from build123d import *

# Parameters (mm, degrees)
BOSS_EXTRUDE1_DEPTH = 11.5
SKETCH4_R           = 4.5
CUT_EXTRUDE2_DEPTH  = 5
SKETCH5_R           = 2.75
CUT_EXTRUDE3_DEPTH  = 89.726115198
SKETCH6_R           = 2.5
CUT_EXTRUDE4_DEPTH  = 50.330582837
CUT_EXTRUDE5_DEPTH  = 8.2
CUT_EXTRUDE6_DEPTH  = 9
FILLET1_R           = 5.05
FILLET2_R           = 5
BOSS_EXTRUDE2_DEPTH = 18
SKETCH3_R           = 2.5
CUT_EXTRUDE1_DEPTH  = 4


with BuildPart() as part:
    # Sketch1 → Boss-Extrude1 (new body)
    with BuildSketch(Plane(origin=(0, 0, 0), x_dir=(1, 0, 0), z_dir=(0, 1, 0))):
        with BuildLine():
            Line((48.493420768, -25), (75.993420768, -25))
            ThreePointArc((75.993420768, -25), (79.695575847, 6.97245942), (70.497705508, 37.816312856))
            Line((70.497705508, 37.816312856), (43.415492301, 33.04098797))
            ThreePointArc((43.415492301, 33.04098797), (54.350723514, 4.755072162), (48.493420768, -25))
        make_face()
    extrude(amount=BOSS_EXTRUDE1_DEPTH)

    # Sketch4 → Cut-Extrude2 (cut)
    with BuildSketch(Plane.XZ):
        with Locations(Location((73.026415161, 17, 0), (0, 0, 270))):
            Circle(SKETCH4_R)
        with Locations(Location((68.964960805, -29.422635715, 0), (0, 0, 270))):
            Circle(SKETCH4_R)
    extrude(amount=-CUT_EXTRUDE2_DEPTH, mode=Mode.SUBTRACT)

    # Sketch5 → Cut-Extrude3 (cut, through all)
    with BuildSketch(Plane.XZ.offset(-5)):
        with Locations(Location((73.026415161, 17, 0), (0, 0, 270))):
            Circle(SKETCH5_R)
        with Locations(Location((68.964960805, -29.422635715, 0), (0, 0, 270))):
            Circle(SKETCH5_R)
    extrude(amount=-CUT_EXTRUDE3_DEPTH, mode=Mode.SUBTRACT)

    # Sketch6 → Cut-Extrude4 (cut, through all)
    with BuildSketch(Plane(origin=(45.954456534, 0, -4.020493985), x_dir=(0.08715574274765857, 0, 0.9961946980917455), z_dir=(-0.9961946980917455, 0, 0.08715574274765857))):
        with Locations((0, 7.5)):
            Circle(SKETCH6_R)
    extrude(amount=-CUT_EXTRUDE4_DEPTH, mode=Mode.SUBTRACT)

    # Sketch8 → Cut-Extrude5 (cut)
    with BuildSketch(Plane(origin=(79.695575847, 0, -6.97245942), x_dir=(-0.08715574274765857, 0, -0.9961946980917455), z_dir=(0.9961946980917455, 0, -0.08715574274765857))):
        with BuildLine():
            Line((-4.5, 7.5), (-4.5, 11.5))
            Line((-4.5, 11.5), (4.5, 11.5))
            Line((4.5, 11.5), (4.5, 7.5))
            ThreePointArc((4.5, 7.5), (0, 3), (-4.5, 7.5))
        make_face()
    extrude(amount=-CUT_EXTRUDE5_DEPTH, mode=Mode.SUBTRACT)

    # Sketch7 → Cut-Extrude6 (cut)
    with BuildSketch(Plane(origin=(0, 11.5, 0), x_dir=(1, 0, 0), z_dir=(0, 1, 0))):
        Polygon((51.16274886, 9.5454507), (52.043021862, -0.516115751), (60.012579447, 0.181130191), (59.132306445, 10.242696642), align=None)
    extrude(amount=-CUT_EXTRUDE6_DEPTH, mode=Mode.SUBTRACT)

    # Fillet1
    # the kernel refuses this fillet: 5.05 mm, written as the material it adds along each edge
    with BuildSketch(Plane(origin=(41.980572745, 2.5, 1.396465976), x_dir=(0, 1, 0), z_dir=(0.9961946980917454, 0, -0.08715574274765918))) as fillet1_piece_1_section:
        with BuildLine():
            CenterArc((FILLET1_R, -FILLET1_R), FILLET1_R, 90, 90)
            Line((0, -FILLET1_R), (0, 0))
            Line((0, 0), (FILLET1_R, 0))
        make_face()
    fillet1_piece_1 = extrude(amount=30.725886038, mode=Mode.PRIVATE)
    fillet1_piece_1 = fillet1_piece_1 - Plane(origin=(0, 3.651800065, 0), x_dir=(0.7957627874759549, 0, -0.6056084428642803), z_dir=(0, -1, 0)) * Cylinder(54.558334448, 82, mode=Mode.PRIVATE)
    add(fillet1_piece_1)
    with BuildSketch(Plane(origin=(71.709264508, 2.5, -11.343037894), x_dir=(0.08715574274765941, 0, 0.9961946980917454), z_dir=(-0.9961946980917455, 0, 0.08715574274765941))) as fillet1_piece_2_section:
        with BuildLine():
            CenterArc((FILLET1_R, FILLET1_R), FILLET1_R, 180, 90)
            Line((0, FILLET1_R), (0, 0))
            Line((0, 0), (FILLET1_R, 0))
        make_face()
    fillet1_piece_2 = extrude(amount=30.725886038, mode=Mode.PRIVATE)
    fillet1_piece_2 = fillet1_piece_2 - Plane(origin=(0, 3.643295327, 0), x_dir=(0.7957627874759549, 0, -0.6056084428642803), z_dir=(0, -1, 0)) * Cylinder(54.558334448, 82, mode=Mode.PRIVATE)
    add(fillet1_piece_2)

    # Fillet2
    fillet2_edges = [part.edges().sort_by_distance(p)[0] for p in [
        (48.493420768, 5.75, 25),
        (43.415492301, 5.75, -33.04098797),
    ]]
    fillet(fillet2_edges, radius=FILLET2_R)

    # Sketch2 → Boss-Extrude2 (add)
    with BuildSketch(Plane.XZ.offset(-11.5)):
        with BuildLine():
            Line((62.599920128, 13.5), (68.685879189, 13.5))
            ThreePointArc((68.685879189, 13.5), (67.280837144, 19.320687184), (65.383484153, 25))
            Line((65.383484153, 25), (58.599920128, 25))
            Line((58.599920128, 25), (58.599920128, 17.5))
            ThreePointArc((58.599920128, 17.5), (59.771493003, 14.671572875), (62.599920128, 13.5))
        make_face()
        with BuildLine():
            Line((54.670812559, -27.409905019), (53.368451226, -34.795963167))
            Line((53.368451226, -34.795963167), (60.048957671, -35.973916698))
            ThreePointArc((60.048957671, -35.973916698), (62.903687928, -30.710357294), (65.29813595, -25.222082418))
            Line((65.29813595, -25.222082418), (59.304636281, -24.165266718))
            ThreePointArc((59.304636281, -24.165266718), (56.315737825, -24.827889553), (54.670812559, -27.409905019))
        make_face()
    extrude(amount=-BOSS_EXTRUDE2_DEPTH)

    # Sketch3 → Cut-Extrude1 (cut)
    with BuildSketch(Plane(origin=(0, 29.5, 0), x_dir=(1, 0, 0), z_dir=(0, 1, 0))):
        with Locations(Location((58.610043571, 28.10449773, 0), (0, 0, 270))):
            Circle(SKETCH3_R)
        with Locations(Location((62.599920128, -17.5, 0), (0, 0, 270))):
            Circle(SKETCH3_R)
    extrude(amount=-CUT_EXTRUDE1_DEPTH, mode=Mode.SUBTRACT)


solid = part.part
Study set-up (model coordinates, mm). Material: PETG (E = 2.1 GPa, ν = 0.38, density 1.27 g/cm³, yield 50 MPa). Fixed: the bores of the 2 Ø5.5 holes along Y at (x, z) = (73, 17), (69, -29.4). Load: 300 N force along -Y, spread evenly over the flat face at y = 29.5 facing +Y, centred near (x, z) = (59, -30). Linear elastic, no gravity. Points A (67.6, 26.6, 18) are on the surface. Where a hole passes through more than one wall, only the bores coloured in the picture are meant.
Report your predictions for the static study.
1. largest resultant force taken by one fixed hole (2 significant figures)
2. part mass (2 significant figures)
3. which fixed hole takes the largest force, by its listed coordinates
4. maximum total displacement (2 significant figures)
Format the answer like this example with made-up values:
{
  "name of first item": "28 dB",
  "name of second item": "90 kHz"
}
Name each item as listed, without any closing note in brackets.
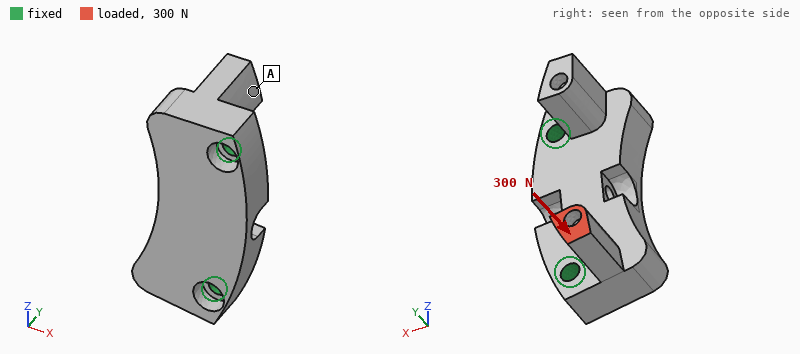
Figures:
{
  "largest resultant force taken by one fixed hole": "300 N",
  "part mass": "24 g",
  "which fixed hole takes the largest force, by its listed coordinates": "(69, -29.4)",
  "maximum total displacement": "0.25 mm"
}
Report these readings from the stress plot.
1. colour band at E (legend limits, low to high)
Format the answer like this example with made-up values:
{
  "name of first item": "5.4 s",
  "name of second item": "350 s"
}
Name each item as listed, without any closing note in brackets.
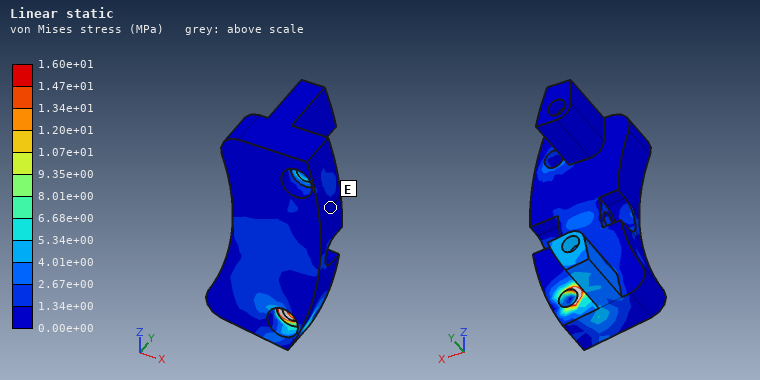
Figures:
{
  "colour band at E": "0.00e+00 to 1.34e+00 MPa"
}
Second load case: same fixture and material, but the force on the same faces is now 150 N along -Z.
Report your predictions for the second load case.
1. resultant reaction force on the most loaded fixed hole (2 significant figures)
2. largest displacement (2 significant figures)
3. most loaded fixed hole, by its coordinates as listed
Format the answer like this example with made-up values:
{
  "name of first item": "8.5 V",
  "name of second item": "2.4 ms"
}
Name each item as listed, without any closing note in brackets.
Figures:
{
  "resultant reaction force on the most loaded fixed hole": "180 N",
  "largest displacement": "0.49 mm",
  "most loaded fixed hole, by its coordinates as listed": "(69, -29.4)"
}
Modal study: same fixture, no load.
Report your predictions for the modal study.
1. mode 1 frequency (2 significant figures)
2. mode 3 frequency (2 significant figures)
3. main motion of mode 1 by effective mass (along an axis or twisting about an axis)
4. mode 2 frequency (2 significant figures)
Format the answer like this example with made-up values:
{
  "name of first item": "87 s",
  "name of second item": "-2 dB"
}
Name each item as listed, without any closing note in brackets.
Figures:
{
  "mode 1 frequency": "1900 Hz",
  "mode 3 frequency": "3000 Hz",
  "main motion of mode 1 by effective mass": "along Y",
  "mode 2 frequency": "2600 Hz"
}
